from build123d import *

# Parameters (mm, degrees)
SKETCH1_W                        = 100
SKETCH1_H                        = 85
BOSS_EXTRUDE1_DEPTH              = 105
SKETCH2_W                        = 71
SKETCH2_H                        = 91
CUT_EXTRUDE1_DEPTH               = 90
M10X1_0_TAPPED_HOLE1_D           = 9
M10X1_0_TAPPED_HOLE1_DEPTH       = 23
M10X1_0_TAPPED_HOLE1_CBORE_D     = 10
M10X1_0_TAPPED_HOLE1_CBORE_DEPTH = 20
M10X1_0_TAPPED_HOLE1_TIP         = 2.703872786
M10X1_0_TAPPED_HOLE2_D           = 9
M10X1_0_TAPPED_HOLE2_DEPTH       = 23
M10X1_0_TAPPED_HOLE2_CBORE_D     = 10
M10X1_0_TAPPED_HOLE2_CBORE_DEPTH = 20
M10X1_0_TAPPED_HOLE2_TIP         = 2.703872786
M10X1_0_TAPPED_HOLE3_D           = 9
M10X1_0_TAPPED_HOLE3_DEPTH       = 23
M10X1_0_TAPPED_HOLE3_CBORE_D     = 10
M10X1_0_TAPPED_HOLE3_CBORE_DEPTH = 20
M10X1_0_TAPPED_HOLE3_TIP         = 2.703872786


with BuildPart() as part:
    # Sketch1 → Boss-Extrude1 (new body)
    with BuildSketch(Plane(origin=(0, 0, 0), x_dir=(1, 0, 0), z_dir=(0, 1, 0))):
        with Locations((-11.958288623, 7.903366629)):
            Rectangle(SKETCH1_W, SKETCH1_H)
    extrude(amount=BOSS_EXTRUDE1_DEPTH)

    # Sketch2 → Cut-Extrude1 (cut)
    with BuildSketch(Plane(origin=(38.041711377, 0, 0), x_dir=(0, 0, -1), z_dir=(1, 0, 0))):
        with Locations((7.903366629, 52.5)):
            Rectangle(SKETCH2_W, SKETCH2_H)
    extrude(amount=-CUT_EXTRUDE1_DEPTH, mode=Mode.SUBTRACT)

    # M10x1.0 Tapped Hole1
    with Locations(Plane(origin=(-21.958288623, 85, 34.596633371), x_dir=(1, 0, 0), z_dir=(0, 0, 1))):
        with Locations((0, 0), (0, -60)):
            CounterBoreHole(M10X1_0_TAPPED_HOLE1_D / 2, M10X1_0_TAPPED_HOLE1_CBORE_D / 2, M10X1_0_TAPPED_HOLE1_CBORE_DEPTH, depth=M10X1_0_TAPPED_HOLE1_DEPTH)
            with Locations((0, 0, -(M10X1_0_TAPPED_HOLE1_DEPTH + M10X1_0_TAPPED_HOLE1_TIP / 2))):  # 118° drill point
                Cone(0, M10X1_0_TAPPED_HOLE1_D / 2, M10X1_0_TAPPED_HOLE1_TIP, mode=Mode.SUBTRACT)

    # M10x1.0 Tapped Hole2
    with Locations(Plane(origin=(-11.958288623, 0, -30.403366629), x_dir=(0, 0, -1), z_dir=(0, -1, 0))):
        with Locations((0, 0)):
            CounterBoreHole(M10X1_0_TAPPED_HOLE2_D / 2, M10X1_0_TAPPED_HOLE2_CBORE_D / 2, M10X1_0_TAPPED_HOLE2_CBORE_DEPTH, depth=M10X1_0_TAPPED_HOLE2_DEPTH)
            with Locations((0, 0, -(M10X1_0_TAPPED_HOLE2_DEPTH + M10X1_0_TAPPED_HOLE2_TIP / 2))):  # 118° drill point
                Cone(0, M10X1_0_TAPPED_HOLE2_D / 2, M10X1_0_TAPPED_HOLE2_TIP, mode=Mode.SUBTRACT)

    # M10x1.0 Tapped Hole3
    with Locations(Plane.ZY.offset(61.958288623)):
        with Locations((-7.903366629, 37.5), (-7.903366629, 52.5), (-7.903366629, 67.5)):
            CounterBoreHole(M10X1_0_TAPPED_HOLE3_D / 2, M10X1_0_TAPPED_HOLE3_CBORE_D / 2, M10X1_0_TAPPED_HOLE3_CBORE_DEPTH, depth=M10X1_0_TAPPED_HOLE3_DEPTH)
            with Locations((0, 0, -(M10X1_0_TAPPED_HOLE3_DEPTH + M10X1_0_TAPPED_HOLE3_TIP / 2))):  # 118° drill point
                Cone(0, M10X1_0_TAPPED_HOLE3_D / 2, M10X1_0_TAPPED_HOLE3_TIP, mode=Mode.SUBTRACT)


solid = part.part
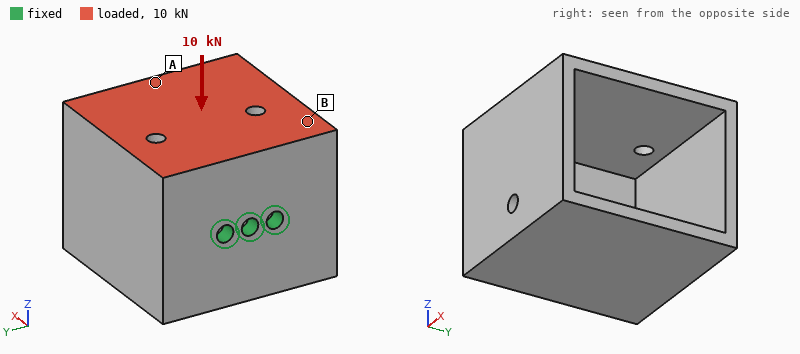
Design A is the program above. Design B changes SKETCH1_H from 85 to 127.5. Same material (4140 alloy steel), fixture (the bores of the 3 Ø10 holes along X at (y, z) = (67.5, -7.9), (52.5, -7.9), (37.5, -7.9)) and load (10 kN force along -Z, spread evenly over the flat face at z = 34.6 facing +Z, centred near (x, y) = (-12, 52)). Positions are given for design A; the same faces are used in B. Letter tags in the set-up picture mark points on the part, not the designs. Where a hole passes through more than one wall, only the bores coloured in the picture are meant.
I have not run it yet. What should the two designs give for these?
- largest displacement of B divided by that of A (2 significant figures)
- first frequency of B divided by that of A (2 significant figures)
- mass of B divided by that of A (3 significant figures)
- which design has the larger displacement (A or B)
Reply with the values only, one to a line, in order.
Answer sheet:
0.75
0.56
2.44
A
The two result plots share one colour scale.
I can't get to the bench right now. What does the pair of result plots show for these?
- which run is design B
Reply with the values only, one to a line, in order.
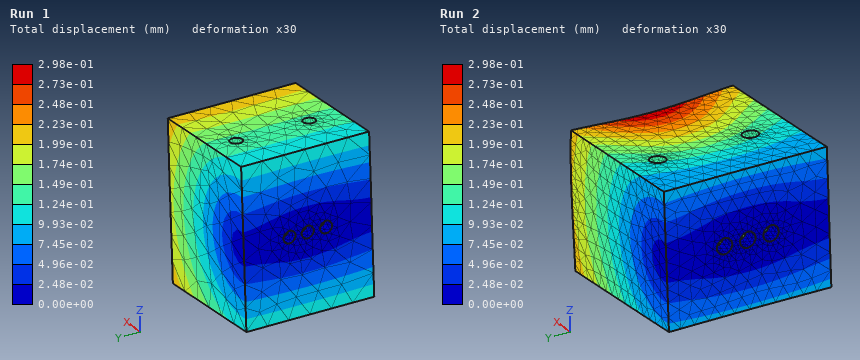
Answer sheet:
Run 1
